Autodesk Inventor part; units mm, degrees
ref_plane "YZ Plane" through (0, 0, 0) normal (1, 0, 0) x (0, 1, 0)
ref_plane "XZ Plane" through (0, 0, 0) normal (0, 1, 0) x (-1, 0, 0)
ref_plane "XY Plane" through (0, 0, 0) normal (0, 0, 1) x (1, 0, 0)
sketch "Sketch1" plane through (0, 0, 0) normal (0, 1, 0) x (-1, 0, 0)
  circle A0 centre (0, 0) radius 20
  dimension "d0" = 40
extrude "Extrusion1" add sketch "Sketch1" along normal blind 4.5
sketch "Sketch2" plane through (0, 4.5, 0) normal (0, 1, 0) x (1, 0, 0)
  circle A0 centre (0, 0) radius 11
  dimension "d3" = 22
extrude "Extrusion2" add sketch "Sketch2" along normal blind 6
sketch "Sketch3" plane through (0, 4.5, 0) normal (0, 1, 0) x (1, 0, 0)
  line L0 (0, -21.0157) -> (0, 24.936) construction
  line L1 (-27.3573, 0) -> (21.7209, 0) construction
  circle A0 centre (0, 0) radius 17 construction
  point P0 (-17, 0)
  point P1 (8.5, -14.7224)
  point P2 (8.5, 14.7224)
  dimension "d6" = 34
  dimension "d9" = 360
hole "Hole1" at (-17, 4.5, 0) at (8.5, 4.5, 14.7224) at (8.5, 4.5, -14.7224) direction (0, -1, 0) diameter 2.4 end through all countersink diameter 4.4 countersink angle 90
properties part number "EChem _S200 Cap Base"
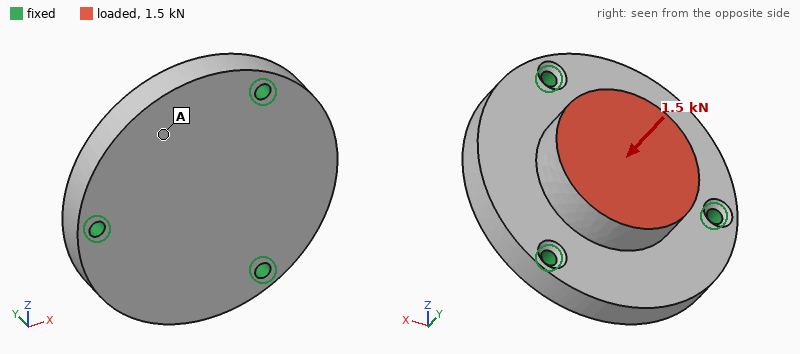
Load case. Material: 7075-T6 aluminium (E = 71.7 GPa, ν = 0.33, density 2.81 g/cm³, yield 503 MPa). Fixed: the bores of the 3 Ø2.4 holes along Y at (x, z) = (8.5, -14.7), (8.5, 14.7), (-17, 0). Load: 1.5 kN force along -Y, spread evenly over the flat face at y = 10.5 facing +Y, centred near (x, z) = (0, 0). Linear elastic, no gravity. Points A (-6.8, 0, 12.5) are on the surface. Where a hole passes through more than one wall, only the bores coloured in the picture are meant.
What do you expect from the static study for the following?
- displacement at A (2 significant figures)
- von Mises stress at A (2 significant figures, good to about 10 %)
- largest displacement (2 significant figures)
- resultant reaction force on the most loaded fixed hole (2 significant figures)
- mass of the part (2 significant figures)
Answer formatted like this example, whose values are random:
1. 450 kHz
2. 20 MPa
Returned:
1. 7.5 µm
2. 12 MPa
3. 8.6 µm
4. 550 N
5. 22 g
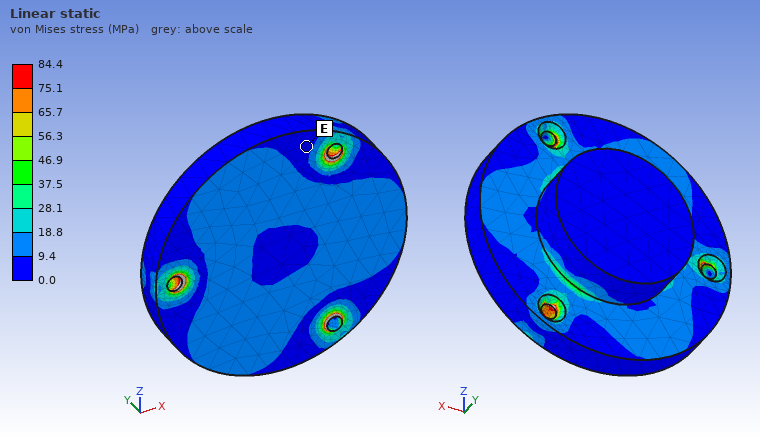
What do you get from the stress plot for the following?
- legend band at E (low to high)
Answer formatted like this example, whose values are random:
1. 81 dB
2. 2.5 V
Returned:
1. 0.0 to 9.4 MPa
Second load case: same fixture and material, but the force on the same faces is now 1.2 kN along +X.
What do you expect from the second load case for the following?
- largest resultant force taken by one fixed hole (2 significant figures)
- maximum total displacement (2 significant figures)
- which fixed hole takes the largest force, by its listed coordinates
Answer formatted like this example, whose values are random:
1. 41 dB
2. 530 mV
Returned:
1. 670 N
2. 9.3 µm
3. (-17, 0)
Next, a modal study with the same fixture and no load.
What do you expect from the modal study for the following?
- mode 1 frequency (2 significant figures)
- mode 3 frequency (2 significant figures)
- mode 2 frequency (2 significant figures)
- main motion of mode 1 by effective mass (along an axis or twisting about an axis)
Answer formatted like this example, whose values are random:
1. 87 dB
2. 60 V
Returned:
1. 16 kHz
2. 18 kHz
3. 18 kHz
4. along Y
